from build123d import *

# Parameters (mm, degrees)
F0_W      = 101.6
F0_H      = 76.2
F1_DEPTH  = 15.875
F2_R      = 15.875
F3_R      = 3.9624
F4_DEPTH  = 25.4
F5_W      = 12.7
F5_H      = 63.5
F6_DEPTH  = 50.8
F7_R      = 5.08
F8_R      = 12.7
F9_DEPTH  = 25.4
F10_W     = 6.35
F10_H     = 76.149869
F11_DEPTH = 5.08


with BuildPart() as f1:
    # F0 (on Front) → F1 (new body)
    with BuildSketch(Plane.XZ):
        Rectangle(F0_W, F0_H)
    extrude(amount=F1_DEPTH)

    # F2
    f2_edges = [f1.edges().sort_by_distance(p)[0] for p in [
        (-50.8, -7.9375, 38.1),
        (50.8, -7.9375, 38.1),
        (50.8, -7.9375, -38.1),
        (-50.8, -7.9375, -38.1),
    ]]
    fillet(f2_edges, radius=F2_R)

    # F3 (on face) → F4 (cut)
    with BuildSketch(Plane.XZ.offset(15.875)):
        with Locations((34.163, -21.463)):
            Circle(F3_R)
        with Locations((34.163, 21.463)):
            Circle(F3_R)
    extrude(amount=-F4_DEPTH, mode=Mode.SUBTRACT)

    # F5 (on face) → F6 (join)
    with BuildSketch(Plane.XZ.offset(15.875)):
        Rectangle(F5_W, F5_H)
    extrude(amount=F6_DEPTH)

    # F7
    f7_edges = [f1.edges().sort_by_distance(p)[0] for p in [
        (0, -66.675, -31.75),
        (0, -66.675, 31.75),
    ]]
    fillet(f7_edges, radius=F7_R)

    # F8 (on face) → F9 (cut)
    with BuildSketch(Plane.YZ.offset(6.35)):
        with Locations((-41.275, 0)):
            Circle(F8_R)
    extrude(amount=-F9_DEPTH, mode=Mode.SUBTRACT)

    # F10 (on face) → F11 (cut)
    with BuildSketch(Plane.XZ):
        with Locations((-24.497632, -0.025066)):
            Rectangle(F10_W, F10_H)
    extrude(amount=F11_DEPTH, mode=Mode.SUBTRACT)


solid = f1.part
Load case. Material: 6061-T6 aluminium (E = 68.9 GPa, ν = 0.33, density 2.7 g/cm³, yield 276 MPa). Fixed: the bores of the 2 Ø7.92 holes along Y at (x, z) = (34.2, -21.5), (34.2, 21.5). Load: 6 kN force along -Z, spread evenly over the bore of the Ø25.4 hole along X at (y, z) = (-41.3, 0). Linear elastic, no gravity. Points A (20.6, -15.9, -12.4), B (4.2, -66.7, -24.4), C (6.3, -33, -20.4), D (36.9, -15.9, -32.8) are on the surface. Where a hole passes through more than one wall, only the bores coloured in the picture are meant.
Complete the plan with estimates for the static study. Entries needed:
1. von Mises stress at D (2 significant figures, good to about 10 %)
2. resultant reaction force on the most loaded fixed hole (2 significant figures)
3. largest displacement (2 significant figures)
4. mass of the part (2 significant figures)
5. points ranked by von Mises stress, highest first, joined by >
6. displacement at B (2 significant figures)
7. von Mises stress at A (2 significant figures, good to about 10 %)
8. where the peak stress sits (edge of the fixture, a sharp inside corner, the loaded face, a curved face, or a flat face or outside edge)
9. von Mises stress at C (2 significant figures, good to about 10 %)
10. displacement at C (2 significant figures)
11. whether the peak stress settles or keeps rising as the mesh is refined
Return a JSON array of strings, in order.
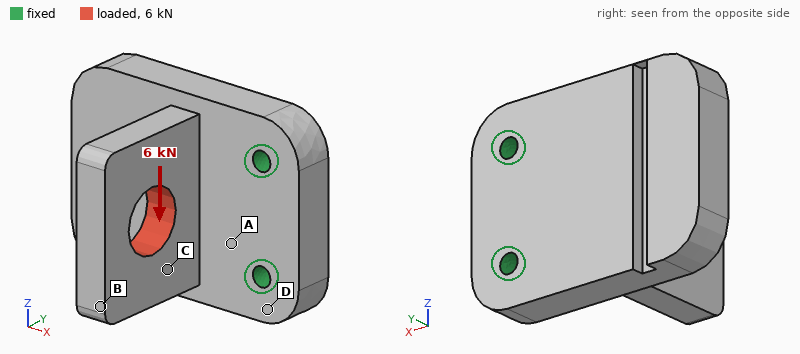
["12 MPa", "6.3 kN", "0.12 mm", "400 g", "A > C > D > B", "0.12 mm", "37 MPa", "edge of the fixture", "22 MPa", "0.057 mm", "keeps rising"]
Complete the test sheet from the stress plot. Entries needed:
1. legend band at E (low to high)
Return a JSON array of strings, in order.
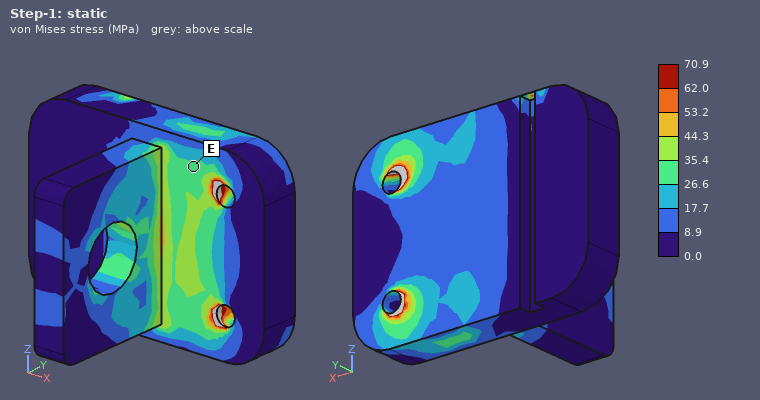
["26.6 to 35.4 MPa"]
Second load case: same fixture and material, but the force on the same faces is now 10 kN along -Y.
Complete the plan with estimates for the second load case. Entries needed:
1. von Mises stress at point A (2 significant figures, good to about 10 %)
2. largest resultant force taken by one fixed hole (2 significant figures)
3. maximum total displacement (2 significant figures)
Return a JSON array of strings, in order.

["56 MPa", "5.0 kN", "0.29 mm"]
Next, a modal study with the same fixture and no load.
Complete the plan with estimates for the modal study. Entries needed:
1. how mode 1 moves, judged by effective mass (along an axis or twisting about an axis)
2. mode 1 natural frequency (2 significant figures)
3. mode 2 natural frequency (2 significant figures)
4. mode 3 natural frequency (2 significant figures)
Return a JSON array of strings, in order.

["along Y", "1500 Hz", "3400 Hz", "3600 Hz"]
